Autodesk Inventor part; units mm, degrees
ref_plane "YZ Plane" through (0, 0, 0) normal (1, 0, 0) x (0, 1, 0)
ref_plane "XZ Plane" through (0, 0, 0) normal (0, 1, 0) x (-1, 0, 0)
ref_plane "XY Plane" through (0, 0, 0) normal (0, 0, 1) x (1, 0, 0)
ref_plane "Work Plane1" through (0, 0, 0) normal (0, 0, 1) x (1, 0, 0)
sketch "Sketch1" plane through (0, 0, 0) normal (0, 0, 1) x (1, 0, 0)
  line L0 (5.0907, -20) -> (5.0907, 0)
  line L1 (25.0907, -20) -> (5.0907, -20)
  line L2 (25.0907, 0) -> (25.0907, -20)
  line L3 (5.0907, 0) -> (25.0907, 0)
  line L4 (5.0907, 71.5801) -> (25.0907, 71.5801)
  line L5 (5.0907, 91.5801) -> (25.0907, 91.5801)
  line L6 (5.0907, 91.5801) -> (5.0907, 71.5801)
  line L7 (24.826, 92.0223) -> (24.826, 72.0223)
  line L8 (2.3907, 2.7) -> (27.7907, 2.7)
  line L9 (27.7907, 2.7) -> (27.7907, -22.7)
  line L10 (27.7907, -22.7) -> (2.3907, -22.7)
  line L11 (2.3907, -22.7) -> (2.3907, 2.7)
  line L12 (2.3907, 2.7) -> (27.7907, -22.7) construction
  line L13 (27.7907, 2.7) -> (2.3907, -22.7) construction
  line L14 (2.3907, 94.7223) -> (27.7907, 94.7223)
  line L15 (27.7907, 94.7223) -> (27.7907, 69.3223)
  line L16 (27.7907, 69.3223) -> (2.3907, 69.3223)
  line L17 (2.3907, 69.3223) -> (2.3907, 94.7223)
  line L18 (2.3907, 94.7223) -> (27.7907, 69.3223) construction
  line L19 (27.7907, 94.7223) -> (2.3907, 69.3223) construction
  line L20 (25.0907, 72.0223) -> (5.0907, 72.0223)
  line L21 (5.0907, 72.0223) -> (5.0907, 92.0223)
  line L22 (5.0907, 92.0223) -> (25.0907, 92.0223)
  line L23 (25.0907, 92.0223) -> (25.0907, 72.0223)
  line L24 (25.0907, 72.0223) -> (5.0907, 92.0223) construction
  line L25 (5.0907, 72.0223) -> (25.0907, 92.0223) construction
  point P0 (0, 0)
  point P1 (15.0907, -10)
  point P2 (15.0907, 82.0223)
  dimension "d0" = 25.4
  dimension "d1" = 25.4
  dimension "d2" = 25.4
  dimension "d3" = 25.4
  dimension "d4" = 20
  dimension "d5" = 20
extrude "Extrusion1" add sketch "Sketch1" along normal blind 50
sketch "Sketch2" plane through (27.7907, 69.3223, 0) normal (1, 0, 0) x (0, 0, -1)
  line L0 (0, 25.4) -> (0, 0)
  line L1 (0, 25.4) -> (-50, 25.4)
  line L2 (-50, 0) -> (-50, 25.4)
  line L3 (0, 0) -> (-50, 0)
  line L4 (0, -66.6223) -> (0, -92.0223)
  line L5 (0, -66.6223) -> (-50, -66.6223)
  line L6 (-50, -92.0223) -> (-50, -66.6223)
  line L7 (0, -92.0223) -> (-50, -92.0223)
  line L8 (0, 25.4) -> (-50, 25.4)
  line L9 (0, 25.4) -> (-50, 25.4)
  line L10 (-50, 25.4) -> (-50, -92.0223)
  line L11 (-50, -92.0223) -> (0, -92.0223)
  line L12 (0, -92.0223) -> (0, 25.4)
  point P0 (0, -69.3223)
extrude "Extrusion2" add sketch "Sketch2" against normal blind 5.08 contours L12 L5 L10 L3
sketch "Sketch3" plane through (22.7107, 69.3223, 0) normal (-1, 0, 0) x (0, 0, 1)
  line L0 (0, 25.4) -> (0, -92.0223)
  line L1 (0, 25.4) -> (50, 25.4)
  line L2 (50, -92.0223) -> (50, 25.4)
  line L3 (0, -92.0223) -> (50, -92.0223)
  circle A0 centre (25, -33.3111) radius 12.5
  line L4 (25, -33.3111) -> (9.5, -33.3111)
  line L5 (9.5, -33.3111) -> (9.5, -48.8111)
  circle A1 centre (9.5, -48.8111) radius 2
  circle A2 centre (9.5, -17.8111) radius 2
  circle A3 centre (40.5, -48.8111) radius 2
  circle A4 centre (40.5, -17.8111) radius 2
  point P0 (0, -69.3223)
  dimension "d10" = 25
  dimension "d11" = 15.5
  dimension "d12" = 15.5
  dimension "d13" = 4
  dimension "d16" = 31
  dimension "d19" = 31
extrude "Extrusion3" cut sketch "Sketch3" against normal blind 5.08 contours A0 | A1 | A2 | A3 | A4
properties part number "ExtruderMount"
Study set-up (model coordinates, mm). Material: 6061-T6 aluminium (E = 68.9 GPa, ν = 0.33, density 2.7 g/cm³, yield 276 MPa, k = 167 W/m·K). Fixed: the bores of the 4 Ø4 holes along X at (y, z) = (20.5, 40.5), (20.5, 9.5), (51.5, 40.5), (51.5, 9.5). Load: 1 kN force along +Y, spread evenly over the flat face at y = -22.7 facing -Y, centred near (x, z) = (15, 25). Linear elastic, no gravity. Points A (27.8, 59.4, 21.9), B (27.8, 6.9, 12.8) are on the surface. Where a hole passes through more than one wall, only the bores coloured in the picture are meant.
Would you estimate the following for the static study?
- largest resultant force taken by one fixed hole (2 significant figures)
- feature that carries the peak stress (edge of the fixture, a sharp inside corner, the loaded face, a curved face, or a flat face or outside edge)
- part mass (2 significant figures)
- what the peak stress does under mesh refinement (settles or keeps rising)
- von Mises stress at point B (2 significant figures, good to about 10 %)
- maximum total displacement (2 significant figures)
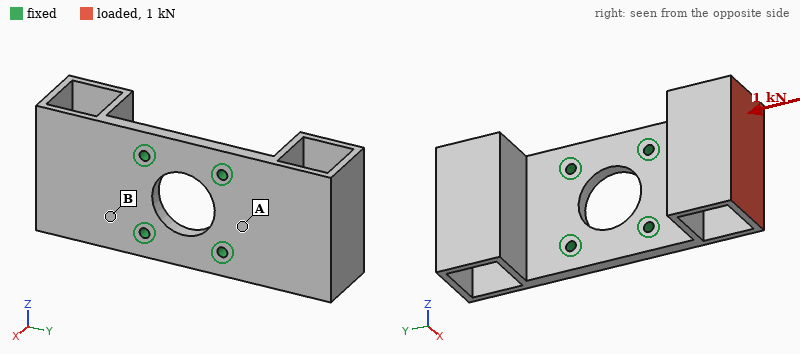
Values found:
470 N
edge of the fixture
100 g
keeps rising
37 MPa
0.37 mm
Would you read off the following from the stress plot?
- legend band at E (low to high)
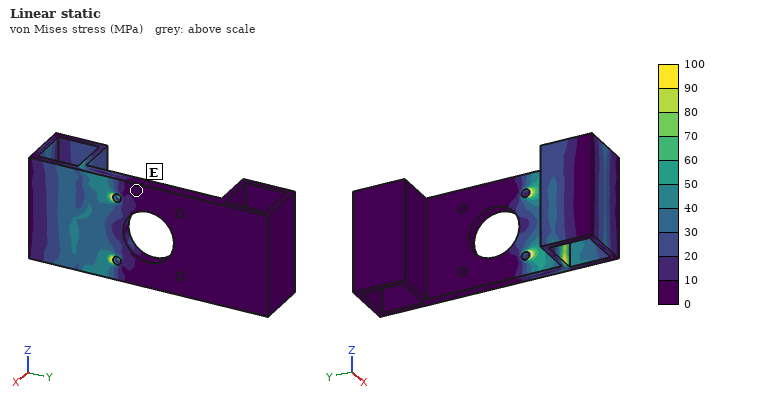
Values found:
0 to 10 MPa
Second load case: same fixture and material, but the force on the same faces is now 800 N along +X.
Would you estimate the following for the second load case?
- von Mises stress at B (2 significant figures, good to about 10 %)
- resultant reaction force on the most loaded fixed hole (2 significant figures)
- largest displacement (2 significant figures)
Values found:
97 MPa
490 N
0.87 mm
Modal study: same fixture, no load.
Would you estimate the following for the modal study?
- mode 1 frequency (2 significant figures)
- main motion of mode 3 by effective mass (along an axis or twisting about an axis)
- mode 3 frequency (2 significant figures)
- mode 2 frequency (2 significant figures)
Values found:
1200 Hz
along Z
3300 Hz
1200 Hz
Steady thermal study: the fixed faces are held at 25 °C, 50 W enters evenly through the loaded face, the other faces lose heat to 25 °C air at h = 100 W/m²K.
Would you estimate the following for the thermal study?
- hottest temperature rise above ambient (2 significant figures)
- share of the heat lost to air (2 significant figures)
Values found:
41 K
46 %
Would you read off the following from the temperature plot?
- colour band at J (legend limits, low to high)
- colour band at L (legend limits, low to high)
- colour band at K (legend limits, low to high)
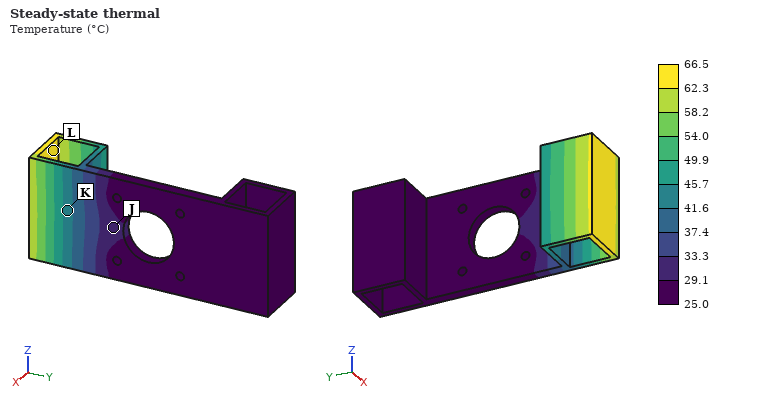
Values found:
29.1 to 33.3 °C
62.3 to 66.5 °C
41.6 to 45.7 °C
